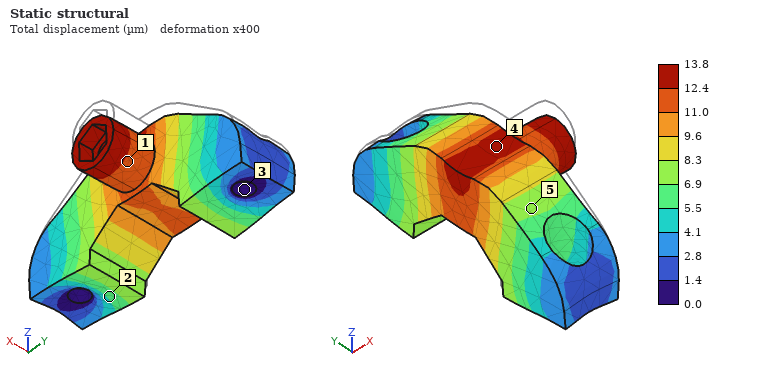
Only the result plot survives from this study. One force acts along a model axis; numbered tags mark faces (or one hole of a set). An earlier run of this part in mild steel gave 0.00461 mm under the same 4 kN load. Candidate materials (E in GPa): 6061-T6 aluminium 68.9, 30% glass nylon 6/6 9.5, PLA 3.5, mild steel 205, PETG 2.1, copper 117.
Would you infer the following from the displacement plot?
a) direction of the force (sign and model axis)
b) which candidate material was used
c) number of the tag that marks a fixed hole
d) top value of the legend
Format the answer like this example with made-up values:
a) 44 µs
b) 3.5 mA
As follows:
a) -Z
b) 6061-T6 aluminium
c) 3
d) 13.8 µm
